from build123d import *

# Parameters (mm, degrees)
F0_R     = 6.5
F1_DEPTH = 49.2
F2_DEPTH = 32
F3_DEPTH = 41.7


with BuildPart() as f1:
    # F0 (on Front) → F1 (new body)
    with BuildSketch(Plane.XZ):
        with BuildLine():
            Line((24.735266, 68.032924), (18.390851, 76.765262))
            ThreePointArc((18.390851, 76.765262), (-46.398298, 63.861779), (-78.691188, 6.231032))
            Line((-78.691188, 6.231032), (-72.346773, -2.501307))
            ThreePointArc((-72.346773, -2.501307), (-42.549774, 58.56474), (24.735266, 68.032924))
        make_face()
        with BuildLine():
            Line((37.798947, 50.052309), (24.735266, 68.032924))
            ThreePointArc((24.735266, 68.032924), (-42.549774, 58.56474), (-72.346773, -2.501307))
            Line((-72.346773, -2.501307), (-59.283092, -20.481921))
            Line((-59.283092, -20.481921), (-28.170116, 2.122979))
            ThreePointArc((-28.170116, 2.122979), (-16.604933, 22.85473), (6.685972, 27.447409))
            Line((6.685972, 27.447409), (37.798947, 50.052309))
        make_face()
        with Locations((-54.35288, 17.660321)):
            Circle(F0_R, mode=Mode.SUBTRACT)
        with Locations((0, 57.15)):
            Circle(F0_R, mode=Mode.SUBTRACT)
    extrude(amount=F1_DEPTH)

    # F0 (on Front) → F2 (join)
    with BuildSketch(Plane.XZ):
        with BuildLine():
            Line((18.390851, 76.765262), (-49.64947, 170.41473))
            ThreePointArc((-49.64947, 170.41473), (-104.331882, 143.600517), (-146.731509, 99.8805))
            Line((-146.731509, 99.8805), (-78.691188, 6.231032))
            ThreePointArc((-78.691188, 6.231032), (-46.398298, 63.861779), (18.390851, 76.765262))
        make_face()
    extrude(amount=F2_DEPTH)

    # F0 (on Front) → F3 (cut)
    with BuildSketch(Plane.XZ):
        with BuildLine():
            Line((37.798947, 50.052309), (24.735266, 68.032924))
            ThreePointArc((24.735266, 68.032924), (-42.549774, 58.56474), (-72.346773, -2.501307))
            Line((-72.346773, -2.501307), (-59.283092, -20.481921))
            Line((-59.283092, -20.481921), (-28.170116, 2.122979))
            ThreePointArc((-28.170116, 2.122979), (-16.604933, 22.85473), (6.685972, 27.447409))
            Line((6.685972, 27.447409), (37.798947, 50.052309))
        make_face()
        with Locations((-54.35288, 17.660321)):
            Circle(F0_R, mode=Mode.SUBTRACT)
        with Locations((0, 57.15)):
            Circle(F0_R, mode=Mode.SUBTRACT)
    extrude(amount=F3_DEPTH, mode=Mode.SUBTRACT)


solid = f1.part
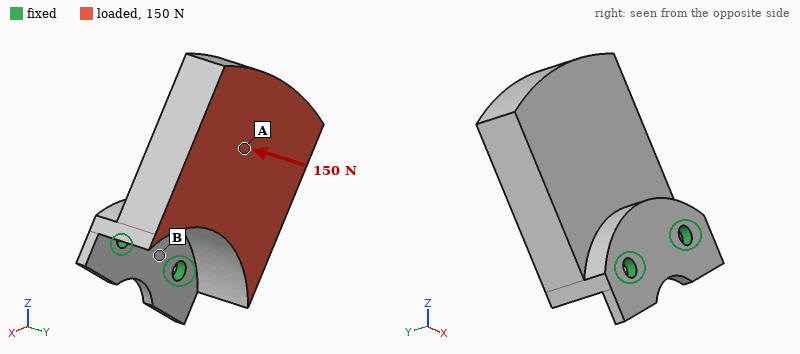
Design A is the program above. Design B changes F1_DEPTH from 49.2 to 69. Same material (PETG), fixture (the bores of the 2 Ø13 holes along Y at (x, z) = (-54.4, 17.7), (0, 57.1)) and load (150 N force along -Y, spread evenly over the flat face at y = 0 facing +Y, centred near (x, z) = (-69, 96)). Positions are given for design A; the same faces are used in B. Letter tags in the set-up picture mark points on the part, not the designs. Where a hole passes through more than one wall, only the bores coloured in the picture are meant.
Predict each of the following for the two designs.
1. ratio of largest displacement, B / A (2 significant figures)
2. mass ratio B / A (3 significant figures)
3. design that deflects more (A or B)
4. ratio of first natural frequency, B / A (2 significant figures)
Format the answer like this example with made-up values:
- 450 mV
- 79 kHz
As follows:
- 0.21
- 1.24
- A
- 2.2
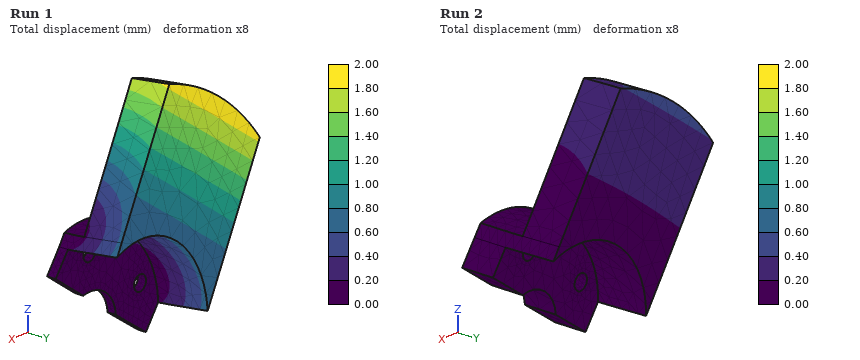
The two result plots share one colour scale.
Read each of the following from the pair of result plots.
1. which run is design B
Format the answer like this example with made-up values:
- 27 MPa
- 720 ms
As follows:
- Run 2
